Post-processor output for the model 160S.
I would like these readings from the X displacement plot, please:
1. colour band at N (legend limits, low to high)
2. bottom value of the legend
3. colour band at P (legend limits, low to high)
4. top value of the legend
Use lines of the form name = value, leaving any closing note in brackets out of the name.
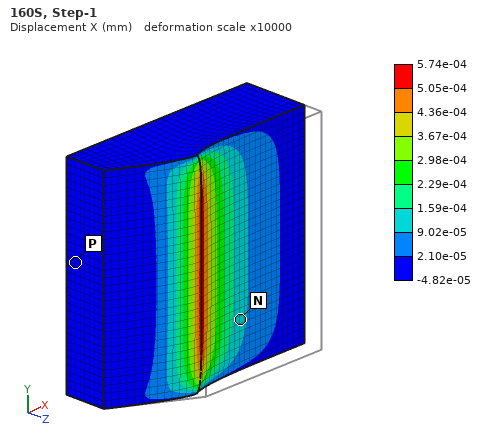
colour band at N = 9.02e-05 to 1.59e-04 mm
bottom value of the legend = -4.82e-05 mm
colour band at P = -4.82e-05 to 2.10e-05 mm
top value of the legend = 5.74e-04 mm
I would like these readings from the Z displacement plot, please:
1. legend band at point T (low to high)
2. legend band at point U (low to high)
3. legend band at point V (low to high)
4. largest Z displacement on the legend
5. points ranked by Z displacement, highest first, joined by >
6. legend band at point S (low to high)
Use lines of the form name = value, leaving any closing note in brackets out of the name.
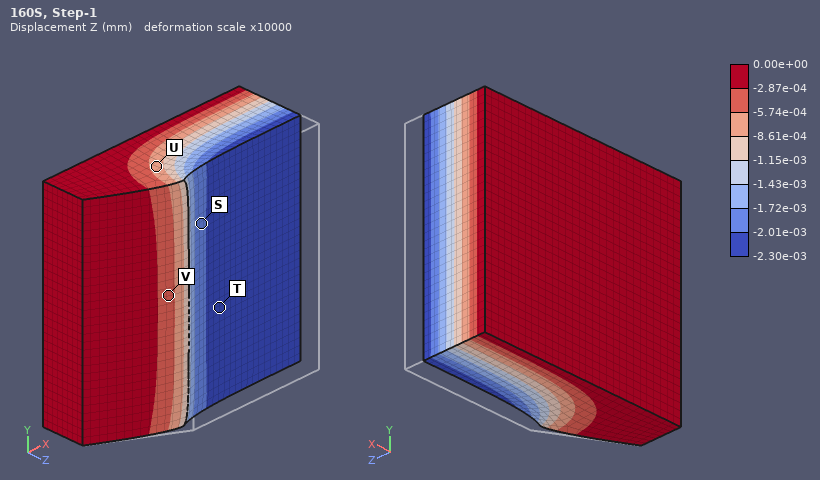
legend band at point T = -2.30e-03 to -2.01e-03 mm
legend band at point U = -8.61e-04 to -5.74e-04 mm
legend band at point V = -5.74e-04 to -2.87e-04 mm
largest Z displacement on the legend = 0.00e+00 mm
points ranked by Z displacement, highest first, joined by > = V > U > S > T
legend band at point S = -2.01e-03 to -1.72e-03 mm
